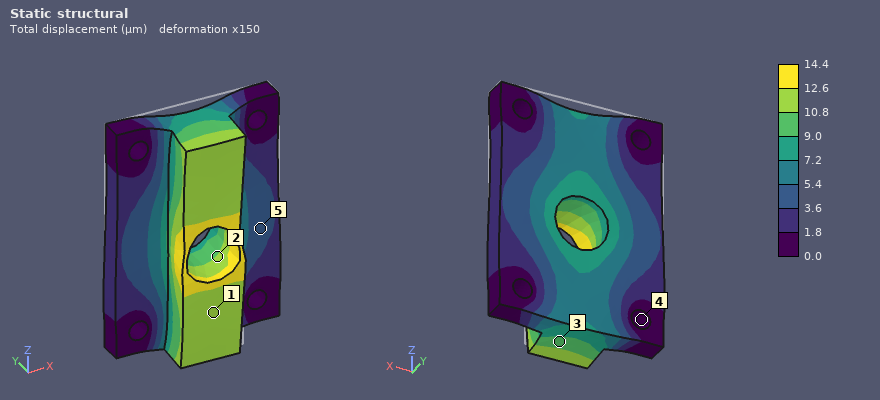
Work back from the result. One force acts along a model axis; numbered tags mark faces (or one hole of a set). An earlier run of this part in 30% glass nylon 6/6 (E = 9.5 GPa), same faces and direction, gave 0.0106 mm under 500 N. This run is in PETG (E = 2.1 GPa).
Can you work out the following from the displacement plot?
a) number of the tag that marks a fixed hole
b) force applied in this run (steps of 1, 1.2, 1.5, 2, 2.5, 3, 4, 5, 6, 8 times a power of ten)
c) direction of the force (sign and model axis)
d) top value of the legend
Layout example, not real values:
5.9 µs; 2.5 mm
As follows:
4; 150 N; -Z; 14.4 µm
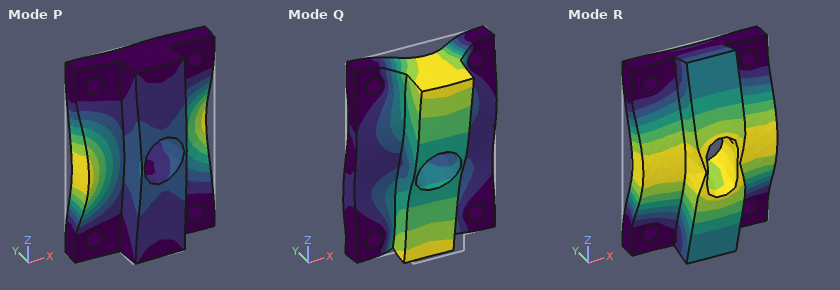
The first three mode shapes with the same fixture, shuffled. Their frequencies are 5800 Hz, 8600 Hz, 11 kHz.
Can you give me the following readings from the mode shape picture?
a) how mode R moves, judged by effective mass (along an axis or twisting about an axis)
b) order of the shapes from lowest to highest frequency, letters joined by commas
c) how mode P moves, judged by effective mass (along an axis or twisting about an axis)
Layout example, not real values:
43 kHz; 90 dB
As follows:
along Y; R, P, Q; twisting about Z
